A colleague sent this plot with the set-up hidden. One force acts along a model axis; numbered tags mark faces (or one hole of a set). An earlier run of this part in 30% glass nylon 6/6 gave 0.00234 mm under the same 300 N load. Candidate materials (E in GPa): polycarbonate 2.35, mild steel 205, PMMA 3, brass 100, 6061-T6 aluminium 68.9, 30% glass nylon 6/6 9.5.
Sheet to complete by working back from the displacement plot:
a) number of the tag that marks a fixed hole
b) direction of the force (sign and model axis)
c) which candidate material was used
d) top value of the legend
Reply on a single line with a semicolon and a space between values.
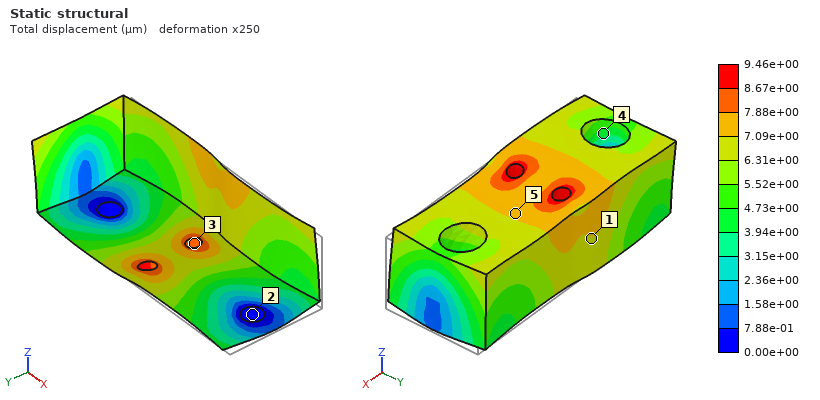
2; -X; polycarbonate; 9.46e+00 µm
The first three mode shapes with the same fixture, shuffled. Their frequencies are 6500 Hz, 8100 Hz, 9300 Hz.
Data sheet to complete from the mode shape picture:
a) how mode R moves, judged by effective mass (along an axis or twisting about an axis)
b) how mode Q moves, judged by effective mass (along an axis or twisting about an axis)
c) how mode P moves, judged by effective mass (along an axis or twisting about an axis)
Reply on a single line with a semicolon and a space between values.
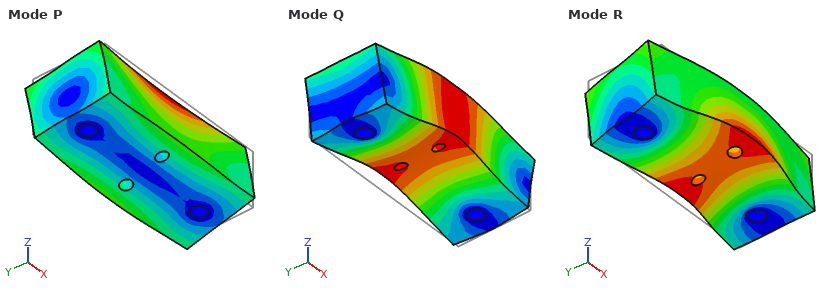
along Y; along Z; along Y
